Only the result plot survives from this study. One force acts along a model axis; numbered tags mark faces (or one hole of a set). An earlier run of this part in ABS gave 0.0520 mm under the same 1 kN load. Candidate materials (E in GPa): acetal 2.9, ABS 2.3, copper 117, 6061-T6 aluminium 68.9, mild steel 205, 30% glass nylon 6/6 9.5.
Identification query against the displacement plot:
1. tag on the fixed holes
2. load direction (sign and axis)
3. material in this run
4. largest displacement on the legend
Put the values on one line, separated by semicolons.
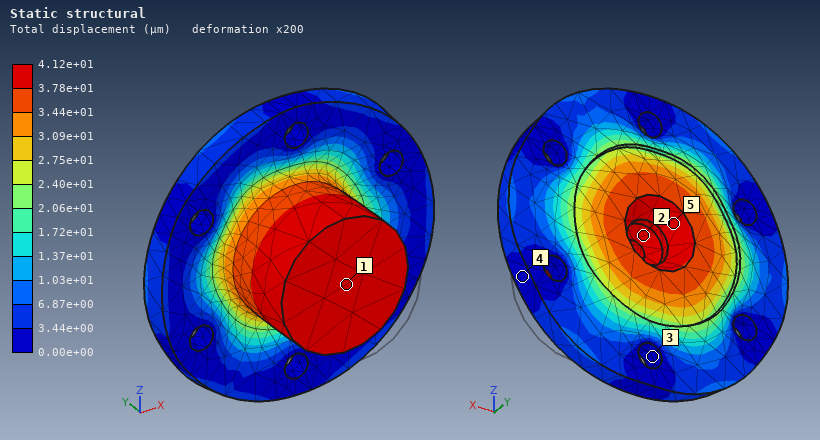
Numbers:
3; +Y; acetal; 4.12e+01 µm
